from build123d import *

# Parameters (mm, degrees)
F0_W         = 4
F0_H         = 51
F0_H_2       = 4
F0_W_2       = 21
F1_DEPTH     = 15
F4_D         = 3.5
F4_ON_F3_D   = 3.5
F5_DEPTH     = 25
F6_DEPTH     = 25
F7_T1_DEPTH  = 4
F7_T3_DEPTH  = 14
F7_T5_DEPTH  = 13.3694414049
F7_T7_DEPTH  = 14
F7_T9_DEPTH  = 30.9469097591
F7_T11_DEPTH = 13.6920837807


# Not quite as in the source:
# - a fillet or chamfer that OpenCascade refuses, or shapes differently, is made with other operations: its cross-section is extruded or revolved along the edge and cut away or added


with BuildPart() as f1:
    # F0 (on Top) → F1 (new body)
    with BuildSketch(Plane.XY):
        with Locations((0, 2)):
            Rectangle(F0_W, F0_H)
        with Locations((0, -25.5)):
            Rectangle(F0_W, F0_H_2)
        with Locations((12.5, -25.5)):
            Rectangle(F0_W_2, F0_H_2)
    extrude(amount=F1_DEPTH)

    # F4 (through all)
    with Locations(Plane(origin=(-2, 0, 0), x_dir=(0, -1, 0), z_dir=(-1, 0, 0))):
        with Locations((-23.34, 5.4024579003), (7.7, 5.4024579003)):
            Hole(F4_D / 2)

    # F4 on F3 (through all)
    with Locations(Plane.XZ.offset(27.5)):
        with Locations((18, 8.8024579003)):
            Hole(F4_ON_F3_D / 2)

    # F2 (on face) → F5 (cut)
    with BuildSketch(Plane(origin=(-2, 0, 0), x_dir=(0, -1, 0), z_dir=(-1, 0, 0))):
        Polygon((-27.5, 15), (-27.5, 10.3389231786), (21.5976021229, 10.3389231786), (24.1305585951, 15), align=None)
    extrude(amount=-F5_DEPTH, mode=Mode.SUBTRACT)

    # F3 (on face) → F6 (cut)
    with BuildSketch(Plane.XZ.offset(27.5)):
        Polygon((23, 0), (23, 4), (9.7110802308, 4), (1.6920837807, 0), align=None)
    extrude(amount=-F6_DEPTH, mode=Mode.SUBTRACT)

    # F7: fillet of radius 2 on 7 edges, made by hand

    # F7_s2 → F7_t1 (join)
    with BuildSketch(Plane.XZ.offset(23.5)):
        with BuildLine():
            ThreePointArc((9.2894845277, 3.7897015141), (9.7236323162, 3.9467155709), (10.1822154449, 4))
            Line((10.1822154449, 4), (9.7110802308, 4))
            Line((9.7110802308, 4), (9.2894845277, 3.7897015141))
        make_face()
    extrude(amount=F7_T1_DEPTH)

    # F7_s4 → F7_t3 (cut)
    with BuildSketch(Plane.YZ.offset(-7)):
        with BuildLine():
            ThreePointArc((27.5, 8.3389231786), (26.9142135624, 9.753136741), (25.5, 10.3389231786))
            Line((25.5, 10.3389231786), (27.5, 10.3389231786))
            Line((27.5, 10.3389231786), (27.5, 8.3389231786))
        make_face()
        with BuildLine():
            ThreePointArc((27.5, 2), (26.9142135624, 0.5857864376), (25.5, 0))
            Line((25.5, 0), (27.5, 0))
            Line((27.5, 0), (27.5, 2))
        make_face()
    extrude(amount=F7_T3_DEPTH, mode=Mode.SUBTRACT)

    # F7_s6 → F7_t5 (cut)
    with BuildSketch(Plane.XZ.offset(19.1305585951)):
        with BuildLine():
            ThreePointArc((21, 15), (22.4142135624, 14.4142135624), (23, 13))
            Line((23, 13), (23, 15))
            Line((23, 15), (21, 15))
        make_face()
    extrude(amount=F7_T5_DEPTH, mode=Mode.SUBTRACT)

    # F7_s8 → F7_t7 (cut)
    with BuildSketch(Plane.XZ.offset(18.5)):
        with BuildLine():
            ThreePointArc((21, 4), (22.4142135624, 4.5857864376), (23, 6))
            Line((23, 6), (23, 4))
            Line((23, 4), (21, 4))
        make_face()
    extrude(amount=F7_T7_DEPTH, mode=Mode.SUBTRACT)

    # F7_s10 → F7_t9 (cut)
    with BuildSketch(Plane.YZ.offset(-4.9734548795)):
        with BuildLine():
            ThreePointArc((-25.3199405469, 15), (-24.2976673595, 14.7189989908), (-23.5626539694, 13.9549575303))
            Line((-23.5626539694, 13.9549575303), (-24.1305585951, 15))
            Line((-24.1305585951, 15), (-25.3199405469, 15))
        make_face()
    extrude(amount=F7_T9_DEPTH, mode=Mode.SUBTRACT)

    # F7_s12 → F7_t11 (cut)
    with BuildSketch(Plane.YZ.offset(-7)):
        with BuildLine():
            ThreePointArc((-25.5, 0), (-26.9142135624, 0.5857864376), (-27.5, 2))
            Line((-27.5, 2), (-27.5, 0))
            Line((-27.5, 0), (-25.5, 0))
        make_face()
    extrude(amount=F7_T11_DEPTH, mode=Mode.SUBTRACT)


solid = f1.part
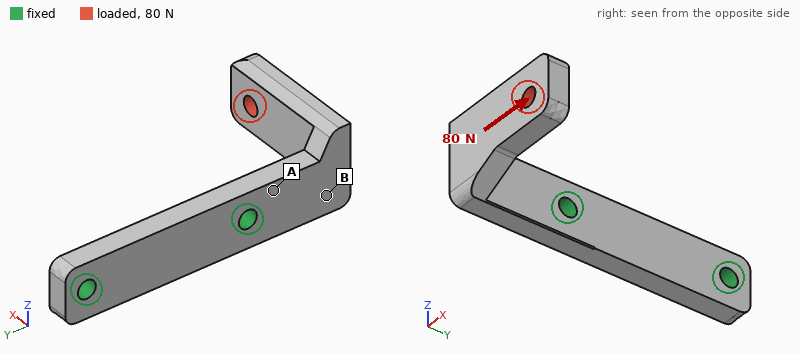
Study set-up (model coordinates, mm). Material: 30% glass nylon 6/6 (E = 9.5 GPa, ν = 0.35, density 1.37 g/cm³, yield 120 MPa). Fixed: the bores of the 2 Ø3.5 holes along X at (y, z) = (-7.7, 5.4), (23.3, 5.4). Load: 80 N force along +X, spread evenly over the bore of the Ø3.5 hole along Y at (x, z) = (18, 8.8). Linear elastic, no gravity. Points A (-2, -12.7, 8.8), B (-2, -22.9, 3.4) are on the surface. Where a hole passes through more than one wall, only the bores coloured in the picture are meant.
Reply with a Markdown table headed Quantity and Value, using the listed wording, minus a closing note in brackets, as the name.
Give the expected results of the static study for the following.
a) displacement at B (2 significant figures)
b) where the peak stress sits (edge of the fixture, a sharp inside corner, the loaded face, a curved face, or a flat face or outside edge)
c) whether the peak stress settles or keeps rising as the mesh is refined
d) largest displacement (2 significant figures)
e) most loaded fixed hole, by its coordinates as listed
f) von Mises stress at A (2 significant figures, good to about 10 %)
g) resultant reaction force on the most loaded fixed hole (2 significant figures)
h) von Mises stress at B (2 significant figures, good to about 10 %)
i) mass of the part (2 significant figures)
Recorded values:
| Quantity | Value |
|---|---|
| displacement at B | 0.20 mm |
| where the peak stress sits | edge of the fixture |
| whether the peak stress settles or keeps rising as the mesh is refined | keeps rising |
| largest displacement | 0.65 mm |
| most loaded fixed hole, by its coordinates as listed | (-7.7, 5.4) |
| von Mises stress at A | 37 MPa |
| resultant reaction force on the most loaded fixed hole | 82 N |
| von Mises stress at B | 9.8 MPa |
| mass of the part | 4.4 g |
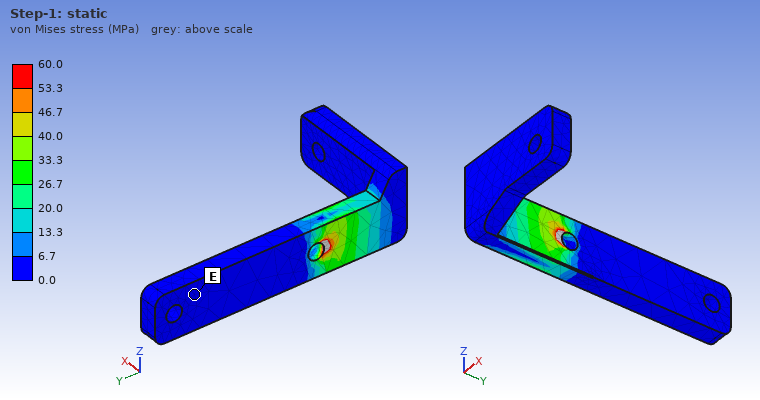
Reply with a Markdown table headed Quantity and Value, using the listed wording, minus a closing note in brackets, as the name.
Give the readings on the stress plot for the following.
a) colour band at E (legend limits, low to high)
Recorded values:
| Quantity | Value |
|---|---|
| colour band at E | 0.0 to 6.7 MPa |
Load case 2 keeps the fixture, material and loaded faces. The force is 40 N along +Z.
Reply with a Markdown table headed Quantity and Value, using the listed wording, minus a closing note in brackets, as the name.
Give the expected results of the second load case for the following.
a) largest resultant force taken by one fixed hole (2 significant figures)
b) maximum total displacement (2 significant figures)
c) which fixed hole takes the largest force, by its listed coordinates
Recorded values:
| Quantity | Value |
|---|---|
| largest resultant force taken by one fixed hole | 49 N |
| maximum total displacement | 0.49 mm |
| which fixed hole takes the largest force, by its listed coordinates | (-7.7, 5.4) |
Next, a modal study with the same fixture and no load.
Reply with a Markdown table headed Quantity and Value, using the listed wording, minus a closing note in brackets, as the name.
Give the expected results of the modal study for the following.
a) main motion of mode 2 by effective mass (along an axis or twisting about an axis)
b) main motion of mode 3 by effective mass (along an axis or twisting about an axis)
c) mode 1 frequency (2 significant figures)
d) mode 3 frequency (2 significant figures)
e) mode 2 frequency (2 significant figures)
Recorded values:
| Quantity | Value |
|---|---|
| main motion of mode 2 by effective mass | along Z |
| main motion of mode 3 by effective mass | along X |
| mode 1 frequency | 1400 Hz |
| mode 3 frequency | 4000 Hz |
| mode 2 frequency | 1800 Hz |
